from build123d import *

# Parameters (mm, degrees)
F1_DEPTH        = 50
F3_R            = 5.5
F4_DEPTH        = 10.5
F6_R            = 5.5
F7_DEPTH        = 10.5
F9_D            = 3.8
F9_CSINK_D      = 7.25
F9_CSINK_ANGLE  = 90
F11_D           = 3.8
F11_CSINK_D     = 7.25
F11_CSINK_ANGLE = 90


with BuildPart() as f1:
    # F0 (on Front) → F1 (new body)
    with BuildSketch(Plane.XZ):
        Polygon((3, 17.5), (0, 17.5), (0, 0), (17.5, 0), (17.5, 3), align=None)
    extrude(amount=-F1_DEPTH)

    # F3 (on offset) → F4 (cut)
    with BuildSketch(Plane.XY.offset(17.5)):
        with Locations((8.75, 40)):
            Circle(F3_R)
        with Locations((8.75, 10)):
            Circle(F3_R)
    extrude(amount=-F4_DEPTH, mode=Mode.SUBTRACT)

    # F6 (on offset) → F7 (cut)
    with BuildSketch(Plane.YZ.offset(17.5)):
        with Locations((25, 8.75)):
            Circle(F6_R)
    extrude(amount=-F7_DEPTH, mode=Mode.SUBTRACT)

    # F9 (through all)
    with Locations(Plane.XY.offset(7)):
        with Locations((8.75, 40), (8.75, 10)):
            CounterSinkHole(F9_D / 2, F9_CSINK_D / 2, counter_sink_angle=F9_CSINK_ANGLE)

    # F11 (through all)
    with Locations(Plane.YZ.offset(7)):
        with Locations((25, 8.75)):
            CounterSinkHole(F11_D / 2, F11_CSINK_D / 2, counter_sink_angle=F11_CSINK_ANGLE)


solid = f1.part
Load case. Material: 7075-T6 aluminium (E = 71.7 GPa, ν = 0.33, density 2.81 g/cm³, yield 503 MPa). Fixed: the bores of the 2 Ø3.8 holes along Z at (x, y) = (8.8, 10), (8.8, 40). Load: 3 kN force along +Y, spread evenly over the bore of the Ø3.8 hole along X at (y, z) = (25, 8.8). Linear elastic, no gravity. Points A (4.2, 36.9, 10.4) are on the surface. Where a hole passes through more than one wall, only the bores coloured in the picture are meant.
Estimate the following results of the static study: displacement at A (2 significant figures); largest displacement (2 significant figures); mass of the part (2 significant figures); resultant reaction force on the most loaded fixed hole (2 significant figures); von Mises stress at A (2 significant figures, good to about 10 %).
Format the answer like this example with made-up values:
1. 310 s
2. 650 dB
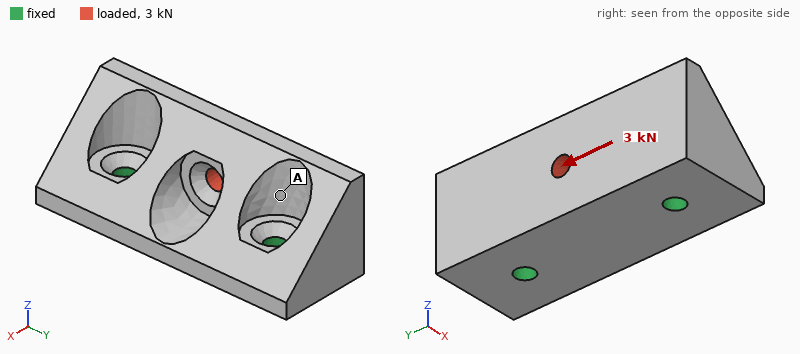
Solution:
1. 5.0 µm
2. 8.4 µm
3. 24 g
4. 1.7 kN
5. 11 MPa
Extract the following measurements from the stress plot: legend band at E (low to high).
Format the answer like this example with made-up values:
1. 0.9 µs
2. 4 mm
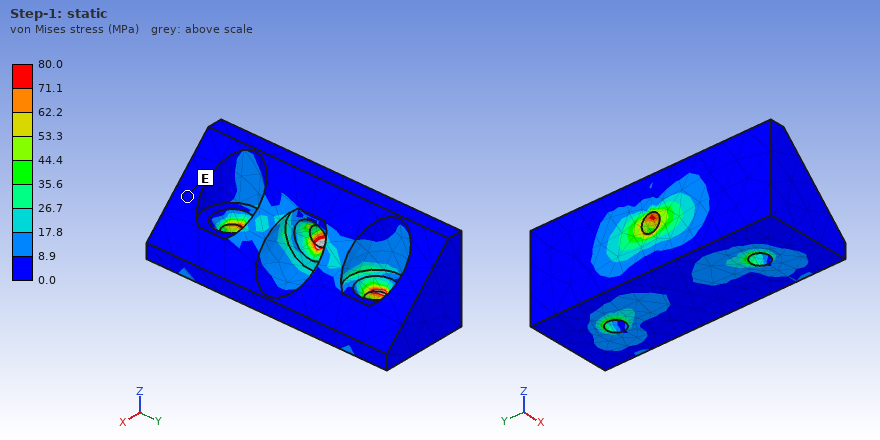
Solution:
1. 0.0 to 8.9 MPa
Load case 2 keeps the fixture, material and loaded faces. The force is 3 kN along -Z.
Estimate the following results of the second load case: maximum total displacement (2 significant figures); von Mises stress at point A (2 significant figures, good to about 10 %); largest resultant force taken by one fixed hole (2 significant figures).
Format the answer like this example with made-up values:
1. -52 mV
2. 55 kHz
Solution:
1. 39 µm
2. 18 MPa
3. 1.6 kN
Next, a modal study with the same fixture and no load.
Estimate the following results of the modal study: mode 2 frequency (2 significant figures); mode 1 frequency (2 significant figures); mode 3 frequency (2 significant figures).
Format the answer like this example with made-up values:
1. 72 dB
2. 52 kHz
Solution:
1. 20 kHz
2. 15 kHz
3. 24 kHz
